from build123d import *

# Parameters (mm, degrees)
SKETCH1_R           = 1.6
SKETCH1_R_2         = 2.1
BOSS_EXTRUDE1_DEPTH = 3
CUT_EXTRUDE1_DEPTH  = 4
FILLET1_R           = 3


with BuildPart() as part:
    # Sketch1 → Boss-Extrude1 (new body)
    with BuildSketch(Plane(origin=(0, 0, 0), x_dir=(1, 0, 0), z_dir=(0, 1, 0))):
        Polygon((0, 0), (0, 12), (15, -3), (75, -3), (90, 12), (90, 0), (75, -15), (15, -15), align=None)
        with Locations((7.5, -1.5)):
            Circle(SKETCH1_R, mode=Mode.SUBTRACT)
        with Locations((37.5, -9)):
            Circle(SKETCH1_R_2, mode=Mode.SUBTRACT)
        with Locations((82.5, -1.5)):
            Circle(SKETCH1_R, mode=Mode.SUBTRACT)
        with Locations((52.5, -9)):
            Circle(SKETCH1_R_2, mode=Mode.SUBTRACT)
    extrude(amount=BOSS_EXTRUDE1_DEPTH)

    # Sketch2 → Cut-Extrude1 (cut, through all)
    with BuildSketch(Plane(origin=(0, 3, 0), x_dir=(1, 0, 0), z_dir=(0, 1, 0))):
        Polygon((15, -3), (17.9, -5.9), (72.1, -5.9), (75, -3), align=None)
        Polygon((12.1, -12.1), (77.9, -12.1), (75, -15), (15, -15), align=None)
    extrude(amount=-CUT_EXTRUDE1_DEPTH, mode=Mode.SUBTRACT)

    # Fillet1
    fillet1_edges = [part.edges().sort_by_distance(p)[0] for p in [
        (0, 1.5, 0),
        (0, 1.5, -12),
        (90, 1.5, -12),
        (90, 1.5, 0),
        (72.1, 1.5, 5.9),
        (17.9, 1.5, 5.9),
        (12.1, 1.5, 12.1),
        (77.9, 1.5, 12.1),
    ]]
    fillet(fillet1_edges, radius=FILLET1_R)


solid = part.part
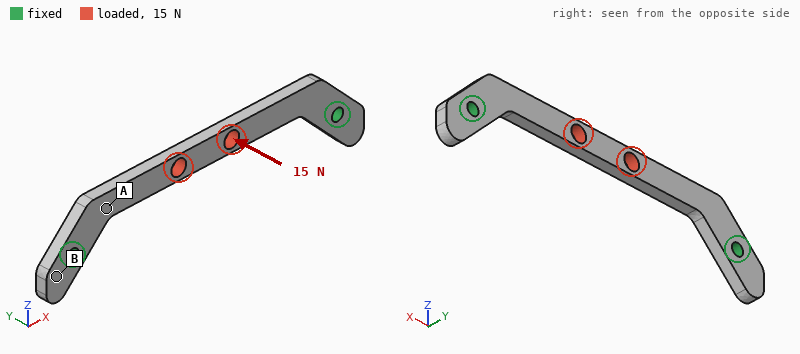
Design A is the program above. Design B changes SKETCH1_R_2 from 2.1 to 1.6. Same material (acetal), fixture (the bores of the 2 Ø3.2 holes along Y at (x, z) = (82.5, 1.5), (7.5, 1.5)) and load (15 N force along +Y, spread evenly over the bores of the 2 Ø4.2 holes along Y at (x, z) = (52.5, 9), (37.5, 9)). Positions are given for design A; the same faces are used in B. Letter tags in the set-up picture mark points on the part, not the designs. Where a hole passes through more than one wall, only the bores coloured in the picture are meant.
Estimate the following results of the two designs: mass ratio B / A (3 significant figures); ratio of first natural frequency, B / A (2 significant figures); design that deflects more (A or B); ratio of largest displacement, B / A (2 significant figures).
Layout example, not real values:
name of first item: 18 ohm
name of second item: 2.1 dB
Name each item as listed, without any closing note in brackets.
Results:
mass ratio B / A: 1.02
ratio of first natural frequency, B / A: 1.0
design that deflects more: A
ratio of largest displacement, B / A: 0.92
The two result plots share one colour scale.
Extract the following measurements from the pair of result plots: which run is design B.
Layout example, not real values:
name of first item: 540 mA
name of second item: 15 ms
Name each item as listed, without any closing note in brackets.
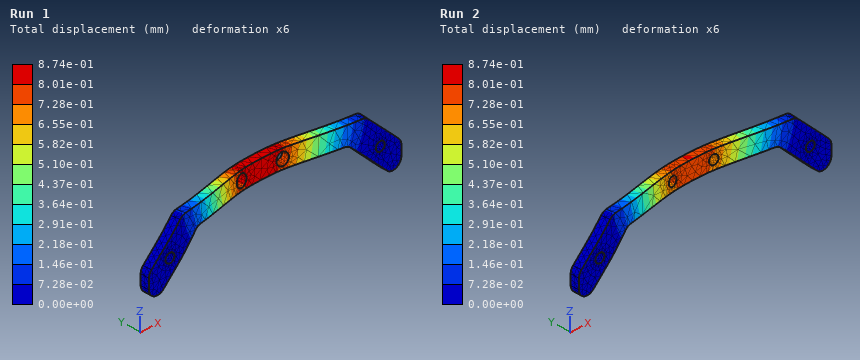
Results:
which run is design B: Run 2
